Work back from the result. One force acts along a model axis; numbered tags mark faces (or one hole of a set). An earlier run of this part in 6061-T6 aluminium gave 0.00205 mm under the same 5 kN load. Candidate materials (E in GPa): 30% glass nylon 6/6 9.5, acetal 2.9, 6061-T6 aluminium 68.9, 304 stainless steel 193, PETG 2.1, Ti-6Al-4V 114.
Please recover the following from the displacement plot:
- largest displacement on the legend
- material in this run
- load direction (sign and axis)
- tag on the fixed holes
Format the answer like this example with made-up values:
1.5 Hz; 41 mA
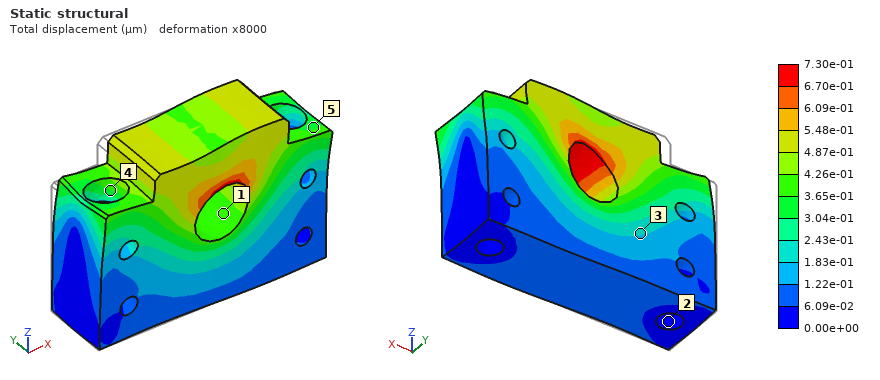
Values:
7.30e-01 µm; 304 stainless steel; +X; 2
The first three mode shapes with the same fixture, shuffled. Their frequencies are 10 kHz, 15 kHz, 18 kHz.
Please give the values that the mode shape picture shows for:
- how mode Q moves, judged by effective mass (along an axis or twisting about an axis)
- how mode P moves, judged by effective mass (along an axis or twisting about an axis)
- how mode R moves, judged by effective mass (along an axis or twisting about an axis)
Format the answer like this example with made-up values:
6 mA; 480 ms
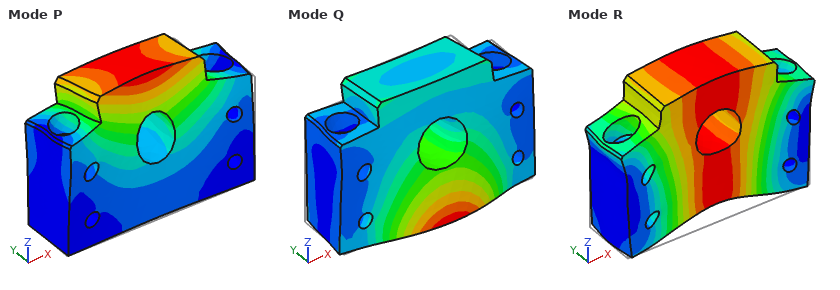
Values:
along Y; along Y; along Z
